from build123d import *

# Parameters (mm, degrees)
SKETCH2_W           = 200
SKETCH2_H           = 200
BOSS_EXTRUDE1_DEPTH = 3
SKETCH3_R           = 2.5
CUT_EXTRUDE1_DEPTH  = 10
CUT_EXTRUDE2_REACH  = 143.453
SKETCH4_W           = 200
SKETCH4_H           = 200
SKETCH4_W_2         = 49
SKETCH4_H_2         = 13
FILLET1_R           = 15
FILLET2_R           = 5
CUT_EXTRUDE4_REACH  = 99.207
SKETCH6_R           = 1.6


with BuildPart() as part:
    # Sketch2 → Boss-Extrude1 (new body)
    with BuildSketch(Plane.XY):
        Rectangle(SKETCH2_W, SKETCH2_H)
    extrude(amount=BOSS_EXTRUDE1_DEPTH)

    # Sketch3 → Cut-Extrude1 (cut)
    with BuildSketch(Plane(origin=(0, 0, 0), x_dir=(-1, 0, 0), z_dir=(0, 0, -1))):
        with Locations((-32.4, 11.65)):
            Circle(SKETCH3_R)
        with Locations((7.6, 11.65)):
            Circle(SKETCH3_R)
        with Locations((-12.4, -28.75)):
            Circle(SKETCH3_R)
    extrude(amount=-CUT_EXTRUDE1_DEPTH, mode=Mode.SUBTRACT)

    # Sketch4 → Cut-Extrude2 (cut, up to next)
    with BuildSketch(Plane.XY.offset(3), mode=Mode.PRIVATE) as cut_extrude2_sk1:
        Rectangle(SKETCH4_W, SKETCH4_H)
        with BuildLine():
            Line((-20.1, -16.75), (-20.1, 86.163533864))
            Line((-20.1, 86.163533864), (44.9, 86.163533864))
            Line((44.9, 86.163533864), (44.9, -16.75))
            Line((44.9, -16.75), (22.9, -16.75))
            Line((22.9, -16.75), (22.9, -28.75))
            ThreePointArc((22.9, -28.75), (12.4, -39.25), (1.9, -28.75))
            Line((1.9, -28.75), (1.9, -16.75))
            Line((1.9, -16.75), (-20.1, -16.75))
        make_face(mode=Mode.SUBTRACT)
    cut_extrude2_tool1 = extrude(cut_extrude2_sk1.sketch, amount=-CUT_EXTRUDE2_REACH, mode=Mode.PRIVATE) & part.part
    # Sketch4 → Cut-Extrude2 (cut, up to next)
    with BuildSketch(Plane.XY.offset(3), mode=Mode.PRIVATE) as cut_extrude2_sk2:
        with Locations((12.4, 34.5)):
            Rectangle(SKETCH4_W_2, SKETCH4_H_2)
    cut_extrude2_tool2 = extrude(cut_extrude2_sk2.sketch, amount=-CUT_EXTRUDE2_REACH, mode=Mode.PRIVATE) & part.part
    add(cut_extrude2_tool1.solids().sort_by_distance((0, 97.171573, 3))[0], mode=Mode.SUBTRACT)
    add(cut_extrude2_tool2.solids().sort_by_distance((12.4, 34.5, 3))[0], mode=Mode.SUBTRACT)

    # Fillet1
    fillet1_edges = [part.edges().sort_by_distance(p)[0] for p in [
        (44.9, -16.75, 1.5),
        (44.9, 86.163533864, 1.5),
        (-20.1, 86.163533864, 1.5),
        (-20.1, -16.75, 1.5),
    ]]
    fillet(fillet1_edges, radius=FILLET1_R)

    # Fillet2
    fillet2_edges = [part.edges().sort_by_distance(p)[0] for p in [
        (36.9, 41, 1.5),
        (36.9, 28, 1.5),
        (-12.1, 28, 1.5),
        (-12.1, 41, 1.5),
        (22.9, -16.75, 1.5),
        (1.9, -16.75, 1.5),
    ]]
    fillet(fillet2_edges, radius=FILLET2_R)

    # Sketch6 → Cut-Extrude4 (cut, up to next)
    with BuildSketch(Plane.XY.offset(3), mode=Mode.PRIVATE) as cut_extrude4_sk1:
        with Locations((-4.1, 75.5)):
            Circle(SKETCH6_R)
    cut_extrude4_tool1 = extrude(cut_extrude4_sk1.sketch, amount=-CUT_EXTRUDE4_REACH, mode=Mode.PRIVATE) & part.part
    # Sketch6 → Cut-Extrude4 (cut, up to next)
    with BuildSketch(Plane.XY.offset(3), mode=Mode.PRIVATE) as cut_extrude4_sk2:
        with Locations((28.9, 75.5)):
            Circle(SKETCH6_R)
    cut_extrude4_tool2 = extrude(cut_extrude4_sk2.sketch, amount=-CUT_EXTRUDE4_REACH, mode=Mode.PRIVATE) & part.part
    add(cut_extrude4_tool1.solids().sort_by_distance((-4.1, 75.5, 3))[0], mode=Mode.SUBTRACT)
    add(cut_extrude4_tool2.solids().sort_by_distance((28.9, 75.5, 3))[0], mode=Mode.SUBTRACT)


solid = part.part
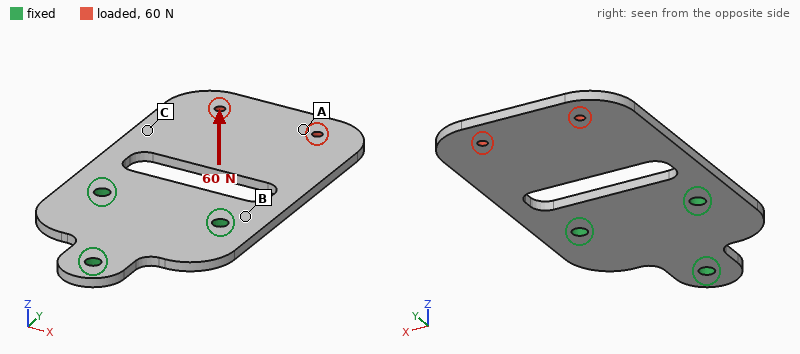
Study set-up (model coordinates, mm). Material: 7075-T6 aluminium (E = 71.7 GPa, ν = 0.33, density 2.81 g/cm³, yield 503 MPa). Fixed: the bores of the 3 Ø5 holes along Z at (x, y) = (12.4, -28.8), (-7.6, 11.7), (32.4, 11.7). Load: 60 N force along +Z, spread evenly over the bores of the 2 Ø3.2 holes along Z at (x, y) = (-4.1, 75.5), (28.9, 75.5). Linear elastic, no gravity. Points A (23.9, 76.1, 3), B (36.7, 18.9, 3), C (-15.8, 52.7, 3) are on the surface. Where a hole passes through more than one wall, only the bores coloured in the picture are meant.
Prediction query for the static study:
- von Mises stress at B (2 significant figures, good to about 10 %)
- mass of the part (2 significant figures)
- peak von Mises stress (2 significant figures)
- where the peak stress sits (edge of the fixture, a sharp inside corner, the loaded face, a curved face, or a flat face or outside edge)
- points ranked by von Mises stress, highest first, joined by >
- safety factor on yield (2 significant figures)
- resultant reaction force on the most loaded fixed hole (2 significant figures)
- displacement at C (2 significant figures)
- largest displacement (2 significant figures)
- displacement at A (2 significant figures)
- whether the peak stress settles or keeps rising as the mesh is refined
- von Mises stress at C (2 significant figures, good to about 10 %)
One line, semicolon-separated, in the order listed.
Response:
50 MPa; 53 g; 130 MPa; a curved face; B > C > A; 3.8; 35 N; 0.54 mm; 1.5 mm; 1.2 mm; settles; 23 MPa
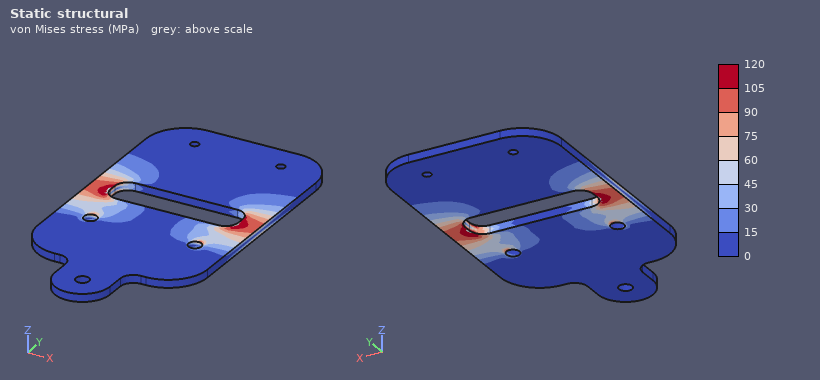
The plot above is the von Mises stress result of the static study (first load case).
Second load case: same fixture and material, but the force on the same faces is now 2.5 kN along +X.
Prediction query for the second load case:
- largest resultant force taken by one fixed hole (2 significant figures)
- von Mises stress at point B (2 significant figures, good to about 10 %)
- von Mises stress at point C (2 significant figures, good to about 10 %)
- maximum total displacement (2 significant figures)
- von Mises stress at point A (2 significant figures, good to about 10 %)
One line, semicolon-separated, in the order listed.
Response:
3.5 kN; 52 MPa; 20 MPa; 0.27 mm; 31 MPa
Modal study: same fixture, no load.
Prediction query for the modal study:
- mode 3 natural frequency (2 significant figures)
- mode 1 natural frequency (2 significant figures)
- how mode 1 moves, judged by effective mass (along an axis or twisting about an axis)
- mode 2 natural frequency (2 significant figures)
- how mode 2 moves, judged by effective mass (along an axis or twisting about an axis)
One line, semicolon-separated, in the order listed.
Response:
2300 Hz; 300 Hz; along Z; 1100 Hz; twisting about Y
